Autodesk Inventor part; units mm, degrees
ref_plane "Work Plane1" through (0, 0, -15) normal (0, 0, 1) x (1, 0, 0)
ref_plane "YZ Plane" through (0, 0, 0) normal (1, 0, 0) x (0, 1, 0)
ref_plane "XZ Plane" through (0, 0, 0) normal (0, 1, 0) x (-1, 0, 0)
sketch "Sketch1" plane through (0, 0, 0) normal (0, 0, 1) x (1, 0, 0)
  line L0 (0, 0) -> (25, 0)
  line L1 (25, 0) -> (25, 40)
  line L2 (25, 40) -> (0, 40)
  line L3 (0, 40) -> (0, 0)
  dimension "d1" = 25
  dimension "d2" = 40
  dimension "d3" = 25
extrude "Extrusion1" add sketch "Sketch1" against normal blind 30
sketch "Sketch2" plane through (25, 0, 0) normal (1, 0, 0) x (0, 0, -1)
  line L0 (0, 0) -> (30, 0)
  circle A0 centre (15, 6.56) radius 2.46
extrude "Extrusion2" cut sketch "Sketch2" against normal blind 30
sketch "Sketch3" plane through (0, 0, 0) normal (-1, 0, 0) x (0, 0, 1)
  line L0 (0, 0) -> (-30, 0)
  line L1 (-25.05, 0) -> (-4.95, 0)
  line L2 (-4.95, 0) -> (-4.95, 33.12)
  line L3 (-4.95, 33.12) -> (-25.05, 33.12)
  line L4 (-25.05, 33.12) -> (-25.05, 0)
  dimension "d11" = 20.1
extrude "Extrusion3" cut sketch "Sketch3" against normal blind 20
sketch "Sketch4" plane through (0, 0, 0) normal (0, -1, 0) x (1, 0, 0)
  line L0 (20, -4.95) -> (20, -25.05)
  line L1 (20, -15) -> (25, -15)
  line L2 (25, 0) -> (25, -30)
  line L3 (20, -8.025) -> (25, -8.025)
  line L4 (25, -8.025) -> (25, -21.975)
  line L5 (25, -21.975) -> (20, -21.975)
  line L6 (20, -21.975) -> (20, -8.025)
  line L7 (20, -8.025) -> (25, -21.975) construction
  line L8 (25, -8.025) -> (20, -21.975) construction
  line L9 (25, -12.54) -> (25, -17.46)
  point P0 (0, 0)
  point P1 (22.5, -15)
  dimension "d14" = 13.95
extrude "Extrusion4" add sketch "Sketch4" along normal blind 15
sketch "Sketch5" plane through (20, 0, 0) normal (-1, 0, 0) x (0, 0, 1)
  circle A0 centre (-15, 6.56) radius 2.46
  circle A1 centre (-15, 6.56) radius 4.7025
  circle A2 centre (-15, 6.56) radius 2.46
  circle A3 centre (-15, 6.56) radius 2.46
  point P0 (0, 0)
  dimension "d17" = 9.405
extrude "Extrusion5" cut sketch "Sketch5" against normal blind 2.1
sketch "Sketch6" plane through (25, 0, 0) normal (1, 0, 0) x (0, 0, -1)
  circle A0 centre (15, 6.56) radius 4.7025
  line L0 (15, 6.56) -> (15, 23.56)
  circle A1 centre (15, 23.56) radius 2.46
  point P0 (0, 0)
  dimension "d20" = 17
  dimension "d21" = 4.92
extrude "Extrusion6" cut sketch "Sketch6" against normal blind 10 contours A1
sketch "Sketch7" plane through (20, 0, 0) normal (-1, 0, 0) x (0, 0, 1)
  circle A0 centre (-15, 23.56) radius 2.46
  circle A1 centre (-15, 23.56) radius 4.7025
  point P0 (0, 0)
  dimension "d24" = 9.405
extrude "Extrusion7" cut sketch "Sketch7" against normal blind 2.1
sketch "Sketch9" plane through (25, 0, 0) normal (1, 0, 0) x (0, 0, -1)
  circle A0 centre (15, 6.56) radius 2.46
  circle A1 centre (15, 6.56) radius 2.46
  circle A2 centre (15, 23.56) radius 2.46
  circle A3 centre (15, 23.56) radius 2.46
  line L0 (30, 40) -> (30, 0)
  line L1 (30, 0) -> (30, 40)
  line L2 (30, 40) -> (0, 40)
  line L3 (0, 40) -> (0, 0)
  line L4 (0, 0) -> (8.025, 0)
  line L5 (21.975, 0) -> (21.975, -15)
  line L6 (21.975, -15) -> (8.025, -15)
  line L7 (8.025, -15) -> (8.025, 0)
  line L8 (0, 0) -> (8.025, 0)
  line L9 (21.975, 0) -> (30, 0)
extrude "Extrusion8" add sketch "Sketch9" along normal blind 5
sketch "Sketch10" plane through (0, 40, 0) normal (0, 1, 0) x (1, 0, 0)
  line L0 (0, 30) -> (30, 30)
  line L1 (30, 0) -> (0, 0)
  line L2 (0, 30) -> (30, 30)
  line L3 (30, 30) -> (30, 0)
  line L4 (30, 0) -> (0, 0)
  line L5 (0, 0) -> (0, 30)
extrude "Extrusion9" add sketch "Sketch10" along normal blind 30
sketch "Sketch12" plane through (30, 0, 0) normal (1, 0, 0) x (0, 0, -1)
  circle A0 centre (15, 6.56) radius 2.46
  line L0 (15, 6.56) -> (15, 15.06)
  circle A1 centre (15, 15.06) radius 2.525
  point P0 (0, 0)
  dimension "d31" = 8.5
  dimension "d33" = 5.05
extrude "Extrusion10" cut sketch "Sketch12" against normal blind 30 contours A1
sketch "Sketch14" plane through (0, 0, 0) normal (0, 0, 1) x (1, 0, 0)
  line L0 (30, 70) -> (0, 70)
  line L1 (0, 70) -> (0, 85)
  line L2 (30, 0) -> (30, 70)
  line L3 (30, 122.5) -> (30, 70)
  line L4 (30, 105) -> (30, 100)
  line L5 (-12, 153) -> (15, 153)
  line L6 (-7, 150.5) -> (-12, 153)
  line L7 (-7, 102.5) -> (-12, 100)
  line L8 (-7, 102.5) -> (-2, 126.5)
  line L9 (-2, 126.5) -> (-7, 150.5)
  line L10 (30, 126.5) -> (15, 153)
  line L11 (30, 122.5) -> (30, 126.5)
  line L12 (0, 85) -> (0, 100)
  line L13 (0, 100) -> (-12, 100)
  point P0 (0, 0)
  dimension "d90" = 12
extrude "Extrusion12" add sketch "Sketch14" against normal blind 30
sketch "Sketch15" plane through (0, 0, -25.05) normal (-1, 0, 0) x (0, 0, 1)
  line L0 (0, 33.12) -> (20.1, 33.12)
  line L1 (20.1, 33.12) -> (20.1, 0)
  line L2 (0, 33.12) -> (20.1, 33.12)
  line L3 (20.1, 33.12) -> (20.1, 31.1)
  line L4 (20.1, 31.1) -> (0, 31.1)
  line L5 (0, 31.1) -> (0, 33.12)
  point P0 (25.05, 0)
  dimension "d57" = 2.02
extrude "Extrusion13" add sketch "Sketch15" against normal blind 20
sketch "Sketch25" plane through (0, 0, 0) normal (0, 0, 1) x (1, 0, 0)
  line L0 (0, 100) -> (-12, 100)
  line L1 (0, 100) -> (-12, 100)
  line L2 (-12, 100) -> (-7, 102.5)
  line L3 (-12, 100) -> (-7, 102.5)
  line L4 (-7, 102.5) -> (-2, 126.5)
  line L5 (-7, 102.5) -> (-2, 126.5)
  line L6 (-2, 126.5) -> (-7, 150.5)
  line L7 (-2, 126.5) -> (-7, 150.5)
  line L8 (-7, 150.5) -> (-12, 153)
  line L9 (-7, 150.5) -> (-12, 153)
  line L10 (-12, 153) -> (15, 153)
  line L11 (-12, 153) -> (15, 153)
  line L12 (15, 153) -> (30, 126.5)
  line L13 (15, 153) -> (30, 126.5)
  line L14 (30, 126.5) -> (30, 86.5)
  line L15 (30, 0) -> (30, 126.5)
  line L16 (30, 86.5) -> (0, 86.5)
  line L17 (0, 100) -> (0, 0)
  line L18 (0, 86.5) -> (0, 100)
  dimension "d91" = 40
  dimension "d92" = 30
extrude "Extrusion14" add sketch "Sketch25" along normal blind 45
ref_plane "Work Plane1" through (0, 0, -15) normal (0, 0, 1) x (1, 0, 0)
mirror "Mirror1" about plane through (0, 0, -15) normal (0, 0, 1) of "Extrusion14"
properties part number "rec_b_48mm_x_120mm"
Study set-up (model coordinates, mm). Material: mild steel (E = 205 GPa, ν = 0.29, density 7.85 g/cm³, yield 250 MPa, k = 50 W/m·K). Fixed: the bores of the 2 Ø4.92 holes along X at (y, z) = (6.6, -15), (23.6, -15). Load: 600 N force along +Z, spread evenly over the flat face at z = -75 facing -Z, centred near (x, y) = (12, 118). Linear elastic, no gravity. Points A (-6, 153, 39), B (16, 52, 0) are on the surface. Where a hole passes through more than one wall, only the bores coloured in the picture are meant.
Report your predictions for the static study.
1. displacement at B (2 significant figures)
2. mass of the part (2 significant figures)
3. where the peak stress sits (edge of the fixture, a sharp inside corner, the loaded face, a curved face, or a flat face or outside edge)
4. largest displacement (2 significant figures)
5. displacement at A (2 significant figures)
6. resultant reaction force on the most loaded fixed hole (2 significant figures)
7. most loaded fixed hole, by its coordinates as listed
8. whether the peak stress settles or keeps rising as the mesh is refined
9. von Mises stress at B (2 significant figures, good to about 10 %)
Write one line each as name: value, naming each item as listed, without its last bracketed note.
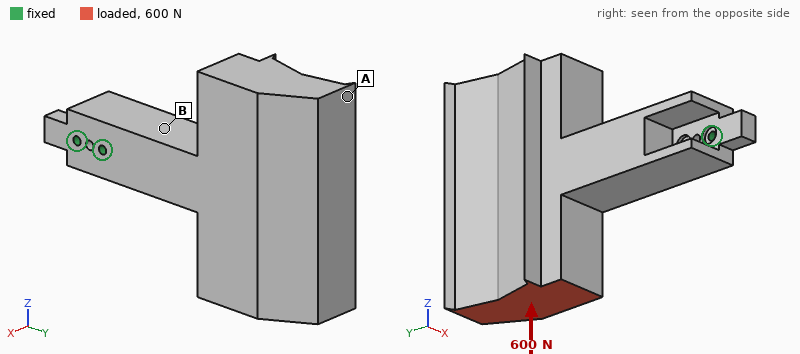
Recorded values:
displacement at B: 11 µm
mass of the part: 2.5 kg
where the peak stress sits: edge of the fixture
largest displacement: 60 µm
displacement at A: 59 µm
resultant reaction force on the most loaded fixed hole: 3.0 kN
most loaded fixed hole, by its coordinates as listed: (23.6, -15)
whether the peak stress settles or keeps rising as the mesh is refined: keeps rising
von Mises stress at B: 9.2 MPa
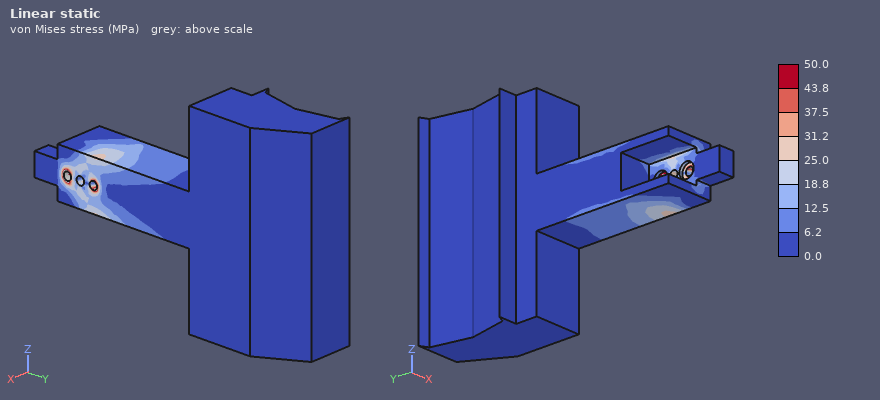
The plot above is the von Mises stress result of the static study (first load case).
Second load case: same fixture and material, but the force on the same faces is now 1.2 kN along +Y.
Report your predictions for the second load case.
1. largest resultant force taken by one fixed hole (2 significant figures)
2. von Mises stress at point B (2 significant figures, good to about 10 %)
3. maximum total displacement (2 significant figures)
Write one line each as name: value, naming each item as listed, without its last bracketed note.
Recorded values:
largest resultant force taken by one fixed hole: 3.3 kN
von Mises stress at point B: 15 MPa
maximum total displacement: 95 µm
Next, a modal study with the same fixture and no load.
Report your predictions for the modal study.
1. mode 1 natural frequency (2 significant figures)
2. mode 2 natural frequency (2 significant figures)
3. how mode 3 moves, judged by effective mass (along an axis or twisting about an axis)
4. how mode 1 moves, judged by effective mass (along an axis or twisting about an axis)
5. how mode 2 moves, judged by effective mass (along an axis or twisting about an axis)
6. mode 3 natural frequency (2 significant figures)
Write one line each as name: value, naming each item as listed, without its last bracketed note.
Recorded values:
mode 1 natural frequency: 380 Hz
mode 2 natural frequency: 410 Hz
how mode 3 moves, judged by effective mass: twisting about Y
how mode 1 moves, judged by effective mass: along X
how mode 2 moves, judged by effective mass: along Z
mode 3 natural frequency: 660 Hz
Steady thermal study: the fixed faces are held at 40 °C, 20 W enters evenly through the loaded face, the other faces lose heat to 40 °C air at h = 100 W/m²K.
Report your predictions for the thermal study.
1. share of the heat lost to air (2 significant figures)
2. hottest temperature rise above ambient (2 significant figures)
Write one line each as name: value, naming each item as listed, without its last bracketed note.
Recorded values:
share of the heat lost to air: 92 %
hottest temperature rise above ambient: 13 K
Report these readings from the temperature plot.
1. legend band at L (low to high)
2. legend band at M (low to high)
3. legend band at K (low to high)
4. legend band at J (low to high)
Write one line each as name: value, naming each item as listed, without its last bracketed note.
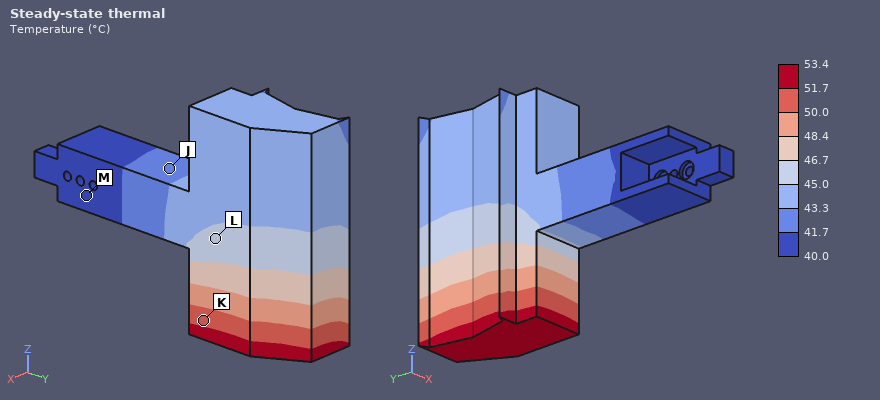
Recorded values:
legend band at L: 45.0 to 46.7 °C
legend band at M: 40.0 to 41.7 °C
legend band at K: 50.0 to 51.7 °C
legend band at J: 41.7 to 43.3 °C
